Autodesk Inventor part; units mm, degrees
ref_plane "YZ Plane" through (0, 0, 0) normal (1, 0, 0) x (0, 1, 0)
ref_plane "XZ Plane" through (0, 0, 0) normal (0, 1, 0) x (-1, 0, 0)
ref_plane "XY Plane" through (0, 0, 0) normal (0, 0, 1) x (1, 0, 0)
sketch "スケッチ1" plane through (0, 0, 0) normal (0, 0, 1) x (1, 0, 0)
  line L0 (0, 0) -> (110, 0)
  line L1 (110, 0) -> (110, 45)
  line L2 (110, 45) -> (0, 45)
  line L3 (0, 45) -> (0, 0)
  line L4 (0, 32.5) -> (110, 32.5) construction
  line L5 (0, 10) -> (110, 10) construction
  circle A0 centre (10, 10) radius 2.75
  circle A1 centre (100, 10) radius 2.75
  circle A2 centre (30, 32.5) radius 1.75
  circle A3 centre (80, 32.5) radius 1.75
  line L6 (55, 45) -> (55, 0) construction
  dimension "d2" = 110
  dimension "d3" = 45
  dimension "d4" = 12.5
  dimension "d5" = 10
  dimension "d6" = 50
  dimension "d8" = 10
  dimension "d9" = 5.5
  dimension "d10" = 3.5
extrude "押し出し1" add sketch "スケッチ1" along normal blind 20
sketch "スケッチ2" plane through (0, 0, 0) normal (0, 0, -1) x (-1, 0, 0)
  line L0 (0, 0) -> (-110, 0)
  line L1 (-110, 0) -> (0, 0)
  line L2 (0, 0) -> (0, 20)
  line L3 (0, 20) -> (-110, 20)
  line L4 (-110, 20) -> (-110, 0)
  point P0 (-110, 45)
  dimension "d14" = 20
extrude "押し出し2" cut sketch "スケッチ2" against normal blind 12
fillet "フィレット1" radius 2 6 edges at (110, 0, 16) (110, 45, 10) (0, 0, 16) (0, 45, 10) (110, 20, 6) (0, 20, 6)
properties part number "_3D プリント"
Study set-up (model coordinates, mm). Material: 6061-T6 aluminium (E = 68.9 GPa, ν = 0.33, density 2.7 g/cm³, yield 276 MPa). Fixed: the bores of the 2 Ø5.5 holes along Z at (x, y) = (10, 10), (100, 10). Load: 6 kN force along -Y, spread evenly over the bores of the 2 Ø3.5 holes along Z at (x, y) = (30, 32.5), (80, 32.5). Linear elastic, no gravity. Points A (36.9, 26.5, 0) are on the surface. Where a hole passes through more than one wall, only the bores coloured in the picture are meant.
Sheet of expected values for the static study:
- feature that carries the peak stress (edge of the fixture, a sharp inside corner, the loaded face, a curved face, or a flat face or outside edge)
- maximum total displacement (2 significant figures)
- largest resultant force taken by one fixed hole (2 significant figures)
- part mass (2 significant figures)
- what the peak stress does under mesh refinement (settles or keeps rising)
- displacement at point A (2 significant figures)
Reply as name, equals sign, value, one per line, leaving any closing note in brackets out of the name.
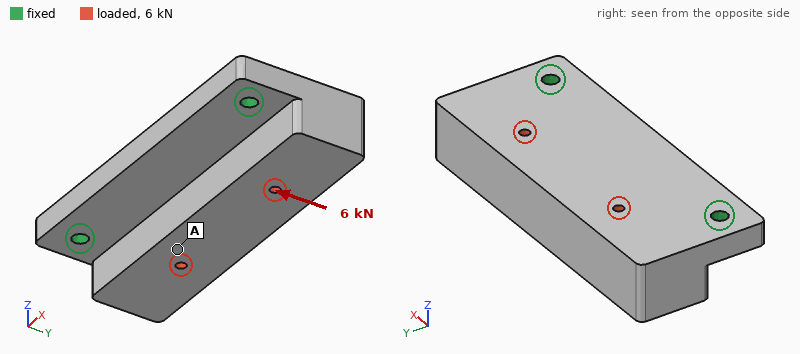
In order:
feature that carries the peak stress = edge of the fixture
maximum total displacement = 0.11 mm
largest resultant force taken by one fixed hole = 3.3 kN
part mass = 190 g
what the peak stress does under mesh refinement = keeps rising
displacement at point A = 0.068 mm
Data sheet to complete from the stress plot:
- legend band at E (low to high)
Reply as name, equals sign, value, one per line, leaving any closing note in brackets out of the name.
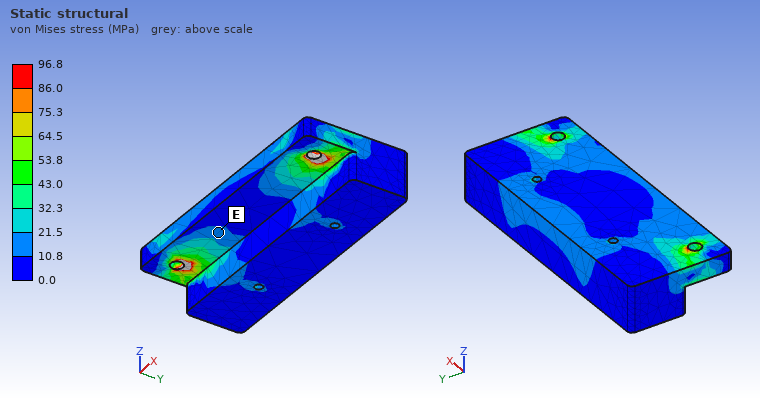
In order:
legend band at E = 10.8 to 21.5 MPa
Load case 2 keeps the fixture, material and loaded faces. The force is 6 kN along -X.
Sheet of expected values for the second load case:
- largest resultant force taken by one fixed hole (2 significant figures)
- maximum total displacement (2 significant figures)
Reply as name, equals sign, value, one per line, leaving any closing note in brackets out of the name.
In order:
largest resultant force taken by one fixed hole = 3.3 kN
maximum total displacement = 12 µm
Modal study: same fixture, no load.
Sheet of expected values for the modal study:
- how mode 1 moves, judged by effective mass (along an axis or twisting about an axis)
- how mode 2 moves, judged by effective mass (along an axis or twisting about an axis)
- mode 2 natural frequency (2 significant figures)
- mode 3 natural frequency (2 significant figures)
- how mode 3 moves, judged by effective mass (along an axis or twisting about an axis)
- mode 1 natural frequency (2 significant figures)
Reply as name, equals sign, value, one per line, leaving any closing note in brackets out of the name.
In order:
how mode 1 moves, judged by effective mass = along Z
how mode 2 moves, judged by effective mass = twisting about Y
mode 2 natural frequency = 6000 Hz
mode 3 natural frequency = 6400 Hz
how mode 3 moves, judged by effective mass = along Z
mode 1 natural frequency = 2200 Hz
